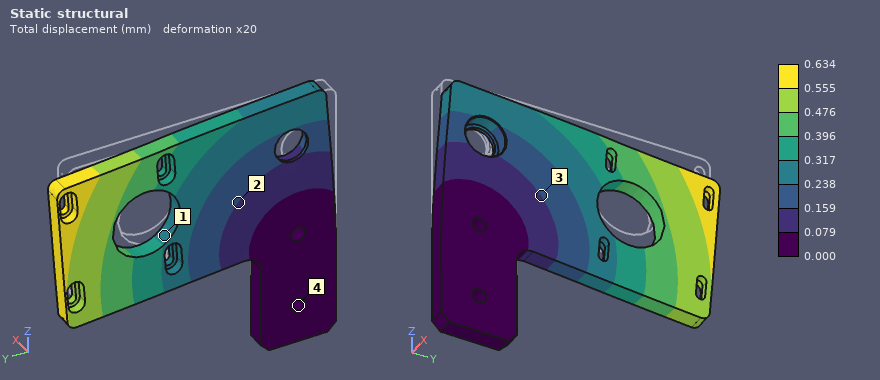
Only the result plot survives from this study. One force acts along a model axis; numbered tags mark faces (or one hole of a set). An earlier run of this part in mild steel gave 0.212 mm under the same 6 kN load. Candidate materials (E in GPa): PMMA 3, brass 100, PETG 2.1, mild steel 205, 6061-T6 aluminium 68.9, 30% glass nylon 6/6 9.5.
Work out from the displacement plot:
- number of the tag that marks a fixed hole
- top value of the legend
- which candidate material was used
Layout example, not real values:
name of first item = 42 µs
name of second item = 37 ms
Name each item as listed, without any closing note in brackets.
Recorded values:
number of the tag that marks a fixed hole = 4
top value of the legend = 0.634 mm
which candidate material was used = 6061-T6 aluminium
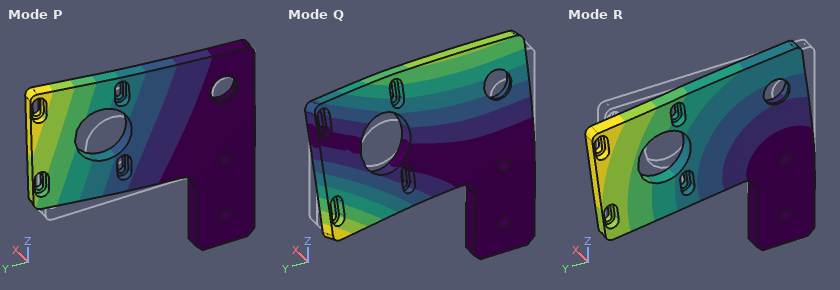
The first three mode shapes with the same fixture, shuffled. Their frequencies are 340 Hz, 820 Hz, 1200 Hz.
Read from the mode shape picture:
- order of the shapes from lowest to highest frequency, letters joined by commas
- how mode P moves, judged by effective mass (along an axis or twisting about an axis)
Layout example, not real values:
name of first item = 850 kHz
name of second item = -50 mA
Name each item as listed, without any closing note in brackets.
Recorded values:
order of the shapes from lowest to highest frequency, letters joined by commas = P, Q, R
how mode P moves, judged by effective mass = along X
